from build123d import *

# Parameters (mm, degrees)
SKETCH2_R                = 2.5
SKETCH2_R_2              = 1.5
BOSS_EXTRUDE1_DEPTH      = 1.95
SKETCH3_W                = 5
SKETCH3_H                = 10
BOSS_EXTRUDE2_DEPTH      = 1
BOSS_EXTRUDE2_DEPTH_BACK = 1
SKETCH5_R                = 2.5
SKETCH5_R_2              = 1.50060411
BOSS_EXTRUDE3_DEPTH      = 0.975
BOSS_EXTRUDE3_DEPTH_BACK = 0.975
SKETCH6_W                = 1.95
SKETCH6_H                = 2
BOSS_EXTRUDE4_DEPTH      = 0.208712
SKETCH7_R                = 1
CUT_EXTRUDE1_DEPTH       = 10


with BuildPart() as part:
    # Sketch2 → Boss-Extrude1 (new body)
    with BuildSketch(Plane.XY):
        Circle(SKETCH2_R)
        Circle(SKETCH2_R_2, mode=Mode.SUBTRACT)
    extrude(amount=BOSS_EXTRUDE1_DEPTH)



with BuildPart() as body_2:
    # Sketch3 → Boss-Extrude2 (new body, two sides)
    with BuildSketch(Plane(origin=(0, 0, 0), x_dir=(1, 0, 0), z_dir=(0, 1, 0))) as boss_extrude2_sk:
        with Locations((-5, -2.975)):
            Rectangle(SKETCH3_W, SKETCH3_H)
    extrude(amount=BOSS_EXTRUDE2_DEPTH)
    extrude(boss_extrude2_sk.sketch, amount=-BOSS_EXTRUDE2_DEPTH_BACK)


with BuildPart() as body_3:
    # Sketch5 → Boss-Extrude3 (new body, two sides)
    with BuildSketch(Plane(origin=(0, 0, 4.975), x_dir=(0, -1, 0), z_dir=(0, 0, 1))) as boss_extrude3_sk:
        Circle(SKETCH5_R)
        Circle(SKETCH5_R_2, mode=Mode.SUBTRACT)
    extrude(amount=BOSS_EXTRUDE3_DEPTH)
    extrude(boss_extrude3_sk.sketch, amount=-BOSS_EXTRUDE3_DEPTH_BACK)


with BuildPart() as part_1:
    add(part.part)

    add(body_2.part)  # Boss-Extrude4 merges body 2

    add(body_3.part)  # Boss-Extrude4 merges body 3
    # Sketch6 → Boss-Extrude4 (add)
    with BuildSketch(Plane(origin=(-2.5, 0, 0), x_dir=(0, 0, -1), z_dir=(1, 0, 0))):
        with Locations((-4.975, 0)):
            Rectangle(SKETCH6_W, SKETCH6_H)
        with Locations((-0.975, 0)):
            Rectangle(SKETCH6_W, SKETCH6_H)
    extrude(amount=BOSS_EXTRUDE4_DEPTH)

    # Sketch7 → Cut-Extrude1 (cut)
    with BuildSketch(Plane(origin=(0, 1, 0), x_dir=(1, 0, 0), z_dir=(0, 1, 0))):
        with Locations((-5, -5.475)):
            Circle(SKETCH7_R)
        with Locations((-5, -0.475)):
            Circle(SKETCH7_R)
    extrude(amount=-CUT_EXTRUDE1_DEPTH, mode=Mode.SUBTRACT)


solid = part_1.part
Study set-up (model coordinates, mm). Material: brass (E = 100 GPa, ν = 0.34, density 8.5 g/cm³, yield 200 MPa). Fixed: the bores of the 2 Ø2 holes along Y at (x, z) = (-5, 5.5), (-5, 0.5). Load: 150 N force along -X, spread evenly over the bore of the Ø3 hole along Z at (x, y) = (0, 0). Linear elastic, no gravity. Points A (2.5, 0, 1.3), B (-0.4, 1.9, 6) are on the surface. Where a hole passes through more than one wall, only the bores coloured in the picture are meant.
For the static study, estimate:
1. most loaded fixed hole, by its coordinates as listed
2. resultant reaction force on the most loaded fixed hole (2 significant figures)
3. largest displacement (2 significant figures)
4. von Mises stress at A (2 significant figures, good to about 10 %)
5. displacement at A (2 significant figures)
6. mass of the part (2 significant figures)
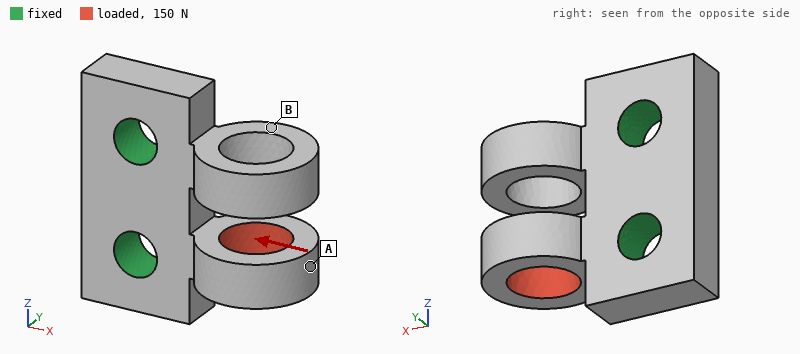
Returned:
(-5, 0.5)
140 N
5.4 µm
48 MPa
5.1 µm
1.2 g
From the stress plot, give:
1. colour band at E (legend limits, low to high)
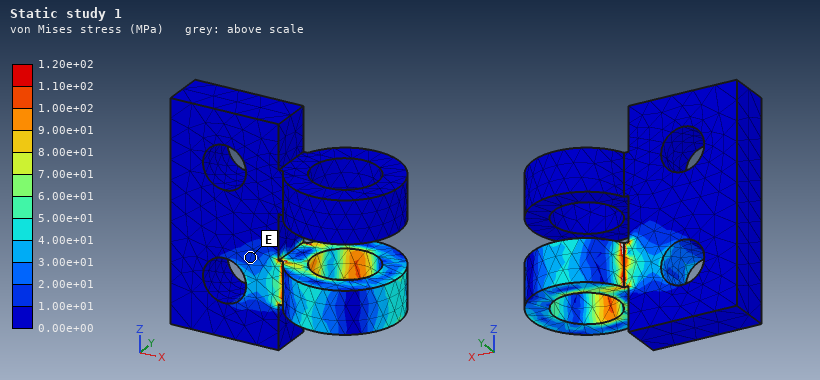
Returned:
1.00e+01 to 2.00e+01 MPa
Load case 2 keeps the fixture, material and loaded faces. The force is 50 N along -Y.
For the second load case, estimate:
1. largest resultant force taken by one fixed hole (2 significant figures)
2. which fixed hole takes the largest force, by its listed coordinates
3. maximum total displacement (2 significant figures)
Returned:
49 N
(-5, 0.5)
21 µm
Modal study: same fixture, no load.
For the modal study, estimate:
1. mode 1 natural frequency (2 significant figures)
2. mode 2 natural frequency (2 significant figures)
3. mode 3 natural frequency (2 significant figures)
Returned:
19 kHz
19 kHz
23 kHz
